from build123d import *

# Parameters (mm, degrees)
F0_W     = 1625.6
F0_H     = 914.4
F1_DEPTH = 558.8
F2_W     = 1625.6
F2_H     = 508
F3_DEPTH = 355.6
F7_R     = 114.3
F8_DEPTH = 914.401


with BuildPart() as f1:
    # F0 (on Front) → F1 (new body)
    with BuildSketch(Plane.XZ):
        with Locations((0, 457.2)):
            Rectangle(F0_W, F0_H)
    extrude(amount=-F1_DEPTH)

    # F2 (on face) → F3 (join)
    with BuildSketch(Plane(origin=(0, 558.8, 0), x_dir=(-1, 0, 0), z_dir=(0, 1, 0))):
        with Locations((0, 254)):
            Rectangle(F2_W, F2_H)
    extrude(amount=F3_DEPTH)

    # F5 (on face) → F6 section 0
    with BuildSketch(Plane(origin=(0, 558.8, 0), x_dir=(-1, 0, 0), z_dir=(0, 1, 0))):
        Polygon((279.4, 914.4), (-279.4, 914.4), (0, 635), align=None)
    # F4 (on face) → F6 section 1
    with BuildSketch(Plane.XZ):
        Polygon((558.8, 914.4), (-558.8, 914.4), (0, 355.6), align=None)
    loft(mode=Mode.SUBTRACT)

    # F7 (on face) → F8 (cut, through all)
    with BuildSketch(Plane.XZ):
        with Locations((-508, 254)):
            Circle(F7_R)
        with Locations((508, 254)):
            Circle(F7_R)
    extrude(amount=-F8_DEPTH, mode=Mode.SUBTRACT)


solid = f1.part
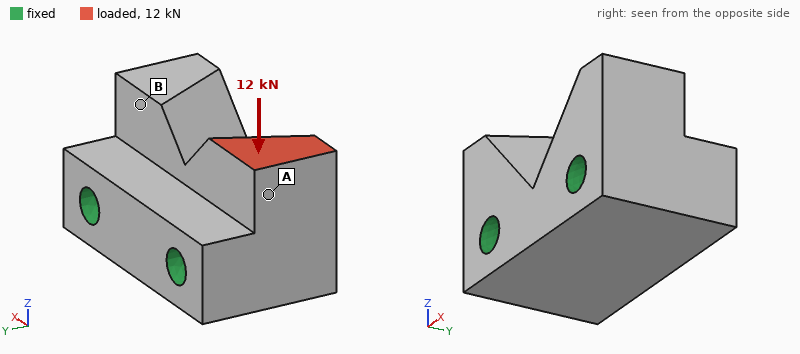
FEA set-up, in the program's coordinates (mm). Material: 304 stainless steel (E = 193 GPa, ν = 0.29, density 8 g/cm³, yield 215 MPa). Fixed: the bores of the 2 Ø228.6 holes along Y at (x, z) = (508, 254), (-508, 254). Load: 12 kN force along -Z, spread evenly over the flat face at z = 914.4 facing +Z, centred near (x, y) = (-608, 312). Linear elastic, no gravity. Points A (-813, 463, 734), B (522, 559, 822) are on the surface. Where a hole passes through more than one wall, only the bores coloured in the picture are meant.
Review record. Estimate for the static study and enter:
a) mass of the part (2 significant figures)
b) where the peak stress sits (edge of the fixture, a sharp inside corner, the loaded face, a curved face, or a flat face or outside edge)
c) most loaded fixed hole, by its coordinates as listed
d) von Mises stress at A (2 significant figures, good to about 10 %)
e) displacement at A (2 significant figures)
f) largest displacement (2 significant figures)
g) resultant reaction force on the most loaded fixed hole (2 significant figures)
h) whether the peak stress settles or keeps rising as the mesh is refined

7600 kg
edge of the fixture
(-508, 254)
0.060 MPa
0.20 µm
0.28 µm
12 kN
keeps rising
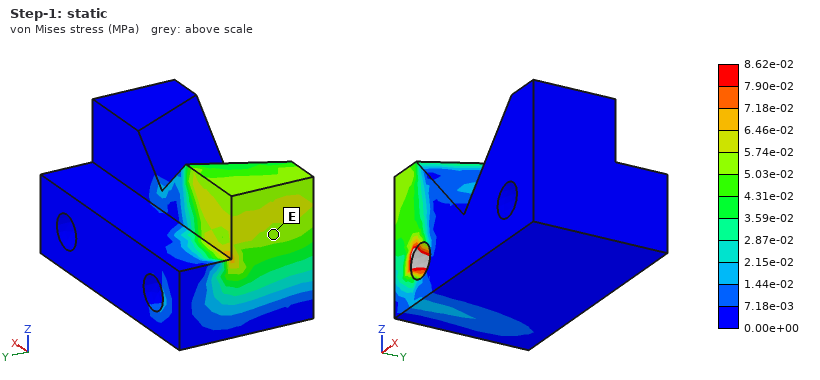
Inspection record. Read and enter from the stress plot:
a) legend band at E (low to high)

5.03e-02 to 5.74e-02 MPa
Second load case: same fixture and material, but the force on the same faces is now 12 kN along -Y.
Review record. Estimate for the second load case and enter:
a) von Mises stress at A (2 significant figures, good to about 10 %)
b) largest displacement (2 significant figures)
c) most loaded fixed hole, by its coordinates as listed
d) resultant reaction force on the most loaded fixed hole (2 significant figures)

0.089 MPa
0.99 µm
(-508, 254)
12 kN
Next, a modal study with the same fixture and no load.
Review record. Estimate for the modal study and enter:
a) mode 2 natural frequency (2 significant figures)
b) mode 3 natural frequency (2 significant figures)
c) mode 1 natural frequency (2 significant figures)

980 Hz
1000 Hz
910 Hz
